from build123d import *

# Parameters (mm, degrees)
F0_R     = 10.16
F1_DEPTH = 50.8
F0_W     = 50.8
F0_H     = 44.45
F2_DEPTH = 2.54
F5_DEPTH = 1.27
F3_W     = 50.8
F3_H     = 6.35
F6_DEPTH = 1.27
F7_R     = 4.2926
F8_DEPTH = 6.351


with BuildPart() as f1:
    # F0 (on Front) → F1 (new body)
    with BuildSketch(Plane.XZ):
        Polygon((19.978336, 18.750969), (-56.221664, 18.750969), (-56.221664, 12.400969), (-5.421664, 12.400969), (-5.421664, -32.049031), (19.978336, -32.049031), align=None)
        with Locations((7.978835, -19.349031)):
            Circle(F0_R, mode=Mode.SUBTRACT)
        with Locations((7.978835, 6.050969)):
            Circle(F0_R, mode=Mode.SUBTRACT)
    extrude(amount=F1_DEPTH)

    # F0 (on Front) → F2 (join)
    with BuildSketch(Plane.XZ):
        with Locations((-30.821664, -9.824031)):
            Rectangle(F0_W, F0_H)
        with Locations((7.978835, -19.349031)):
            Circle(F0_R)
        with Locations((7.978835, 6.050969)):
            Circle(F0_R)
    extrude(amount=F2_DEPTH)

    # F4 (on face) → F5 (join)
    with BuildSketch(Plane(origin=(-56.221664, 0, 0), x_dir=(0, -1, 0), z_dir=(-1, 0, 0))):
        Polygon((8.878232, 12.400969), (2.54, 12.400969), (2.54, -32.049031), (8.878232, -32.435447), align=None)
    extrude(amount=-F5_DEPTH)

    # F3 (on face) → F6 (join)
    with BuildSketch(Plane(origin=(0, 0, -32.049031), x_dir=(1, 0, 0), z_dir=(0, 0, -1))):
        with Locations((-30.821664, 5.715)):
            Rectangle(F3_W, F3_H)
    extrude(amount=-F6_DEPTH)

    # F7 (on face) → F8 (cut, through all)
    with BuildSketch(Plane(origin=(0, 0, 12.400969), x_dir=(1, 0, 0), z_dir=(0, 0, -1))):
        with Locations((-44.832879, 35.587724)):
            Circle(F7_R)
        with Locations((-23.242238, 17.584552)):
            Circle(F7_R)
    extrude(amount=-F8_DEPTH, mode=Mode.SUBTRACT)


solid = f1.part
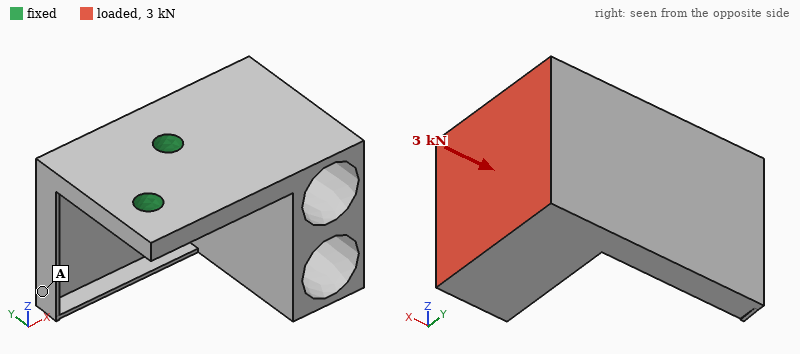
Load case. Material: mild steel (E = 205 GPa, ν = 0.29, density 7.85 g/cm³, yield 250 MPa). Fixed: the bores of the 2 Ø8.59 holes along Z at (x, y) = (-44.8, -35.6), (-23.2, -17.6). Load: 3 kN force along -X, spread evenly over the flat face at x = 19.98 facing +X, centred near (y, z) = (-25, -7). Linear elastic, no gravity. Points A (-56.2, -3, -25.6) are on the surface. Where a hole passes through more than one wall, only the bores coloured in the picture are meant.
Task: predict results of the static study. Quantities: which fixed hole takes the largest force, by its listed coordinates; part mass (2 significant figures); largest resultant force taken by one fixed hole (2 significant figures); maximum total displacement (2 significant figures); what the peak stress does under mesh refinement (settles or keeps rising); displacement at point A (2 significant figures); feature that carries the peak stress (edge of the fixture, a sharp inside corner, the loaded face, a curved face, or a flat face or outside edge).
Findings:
(-23.2, -17.6)
440 g
1.9 kN
0.15 mm
keeps rising
0.13 mm
edge of the fixture
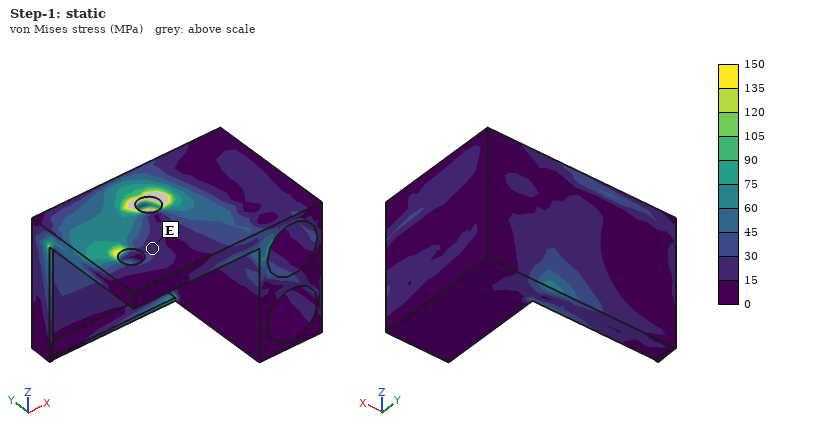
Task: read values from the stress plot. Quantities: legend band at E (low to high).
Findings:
15 to 30 MPa
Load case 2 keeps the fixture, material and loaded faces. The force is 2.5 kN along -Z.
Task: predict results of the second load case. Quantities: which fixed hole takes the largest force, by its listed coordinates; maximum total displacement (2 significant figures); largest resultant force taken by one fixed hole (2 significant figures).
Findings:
(-23.2, -17.6)
0.19 mm
3.6 kN
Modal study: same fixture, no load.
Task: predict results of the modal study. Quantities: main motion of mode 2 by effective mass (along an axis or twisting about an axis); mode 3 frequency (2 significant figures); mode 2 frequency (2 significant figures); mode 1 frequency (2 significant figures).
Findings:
along Y
2800 Hz
1600 Hz
1300 Hz
